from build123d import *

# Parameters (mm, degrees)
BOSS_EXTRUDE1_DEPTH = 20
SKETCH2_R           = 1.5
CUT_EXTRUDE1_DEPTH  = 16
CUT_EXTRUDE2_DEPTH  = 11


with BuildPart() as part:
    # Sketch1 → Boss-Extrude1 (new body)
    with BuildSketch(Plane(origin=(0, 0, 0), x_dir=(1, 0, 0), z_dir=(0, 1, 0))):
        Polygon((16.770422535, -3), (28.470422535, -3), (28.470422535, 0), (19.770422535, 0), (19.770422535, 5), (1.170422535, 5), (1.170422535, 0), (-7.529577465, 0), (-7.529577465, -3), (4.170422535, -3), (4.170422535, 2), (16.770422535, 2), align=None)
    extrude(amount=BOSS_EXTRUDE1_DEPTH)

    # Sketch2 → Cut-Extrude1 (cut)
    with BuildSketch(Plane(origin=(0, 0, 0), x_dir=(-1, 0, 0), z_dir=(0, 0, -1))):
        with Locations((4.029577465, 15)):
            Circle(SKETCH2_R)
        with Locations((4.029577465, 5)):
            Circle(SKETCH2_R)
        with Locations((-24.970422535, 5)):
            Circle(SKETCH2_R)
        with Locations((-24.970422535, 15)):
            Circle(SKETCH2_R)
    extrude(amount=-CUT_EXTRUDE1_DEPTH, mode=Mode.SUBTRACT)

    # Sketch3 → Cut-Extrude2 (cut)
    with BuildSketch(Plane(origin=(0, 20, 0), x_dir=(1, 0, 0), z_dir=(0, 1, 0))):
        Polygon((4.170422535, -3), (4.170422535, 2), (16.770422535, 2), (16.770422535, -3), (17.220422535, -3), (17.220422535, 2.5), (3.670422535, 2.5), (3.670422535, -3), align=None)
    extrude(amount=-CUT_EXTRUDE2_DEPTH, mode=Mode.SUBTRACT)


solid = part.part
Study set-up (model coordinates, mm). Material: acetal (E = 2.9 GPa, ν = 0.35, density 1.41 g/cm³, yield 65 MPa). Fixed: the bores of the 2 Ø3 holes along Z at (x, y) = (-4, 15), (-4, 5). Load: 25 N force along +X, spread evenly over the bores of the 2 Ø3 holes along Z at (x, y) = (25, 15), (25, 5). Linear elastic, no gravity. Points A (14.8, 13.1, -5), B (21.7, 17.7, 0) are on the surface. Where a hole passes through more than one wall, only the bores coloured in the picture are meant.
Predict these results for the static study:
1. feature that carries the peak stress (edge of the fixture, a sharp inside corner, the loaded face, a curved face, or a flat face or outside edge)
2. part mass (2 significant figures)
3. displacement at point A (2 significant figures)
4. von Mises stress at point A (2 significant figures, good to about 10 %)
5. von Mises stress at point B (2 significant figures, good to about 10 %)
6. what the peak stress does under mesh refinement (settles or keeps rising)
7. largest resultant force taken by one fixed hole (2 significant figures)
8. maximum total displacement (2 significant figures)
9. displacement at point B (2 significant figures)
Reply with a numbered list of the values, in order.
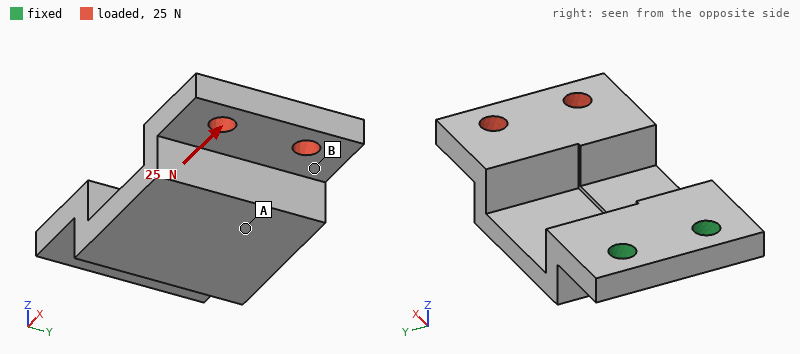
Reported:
1. a sharp inside corner
2. 3.6 g
3. 0.11 mm
4. 3.8 MPa
5. 0.80 MPa
6. keeps rising
7. 13 N
8. 0.44 mm
9. 0.27 mm
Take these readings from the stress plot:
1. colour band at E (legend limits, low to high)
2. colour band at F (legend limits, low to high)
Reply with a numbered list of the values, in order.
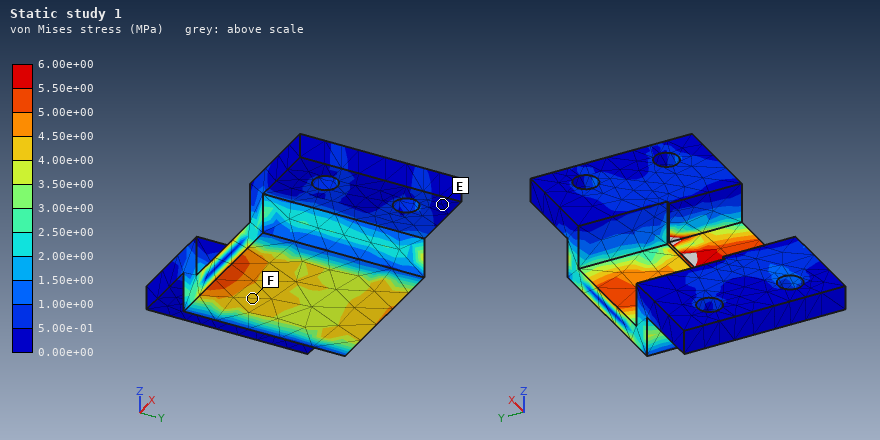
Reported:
1. 0.00e+00 to 5.00e-01 MPa
2. 4.00e+00 to 4.50e+00 MPa
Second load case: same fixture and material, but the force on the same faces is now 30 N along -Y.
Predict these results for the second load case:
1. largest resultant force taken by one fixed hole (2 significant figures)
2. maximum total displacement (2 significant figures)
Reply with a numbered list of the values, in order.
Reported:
1. 72 N
2. 0.50 mm
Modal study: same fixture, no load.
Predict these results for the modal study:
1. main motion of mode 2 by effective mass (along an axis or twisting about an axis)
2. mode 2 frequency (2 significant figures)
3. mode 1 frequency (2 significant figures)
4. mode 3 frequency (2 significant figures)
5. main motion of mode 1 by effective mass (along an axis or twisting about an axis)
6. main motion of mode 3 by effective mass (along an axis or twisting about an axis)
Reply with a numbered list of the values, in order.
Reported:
1. along Y
2. 1300 Hz
3. 550 Hz
4. 2300 Hz
5. along Z
6. along X
